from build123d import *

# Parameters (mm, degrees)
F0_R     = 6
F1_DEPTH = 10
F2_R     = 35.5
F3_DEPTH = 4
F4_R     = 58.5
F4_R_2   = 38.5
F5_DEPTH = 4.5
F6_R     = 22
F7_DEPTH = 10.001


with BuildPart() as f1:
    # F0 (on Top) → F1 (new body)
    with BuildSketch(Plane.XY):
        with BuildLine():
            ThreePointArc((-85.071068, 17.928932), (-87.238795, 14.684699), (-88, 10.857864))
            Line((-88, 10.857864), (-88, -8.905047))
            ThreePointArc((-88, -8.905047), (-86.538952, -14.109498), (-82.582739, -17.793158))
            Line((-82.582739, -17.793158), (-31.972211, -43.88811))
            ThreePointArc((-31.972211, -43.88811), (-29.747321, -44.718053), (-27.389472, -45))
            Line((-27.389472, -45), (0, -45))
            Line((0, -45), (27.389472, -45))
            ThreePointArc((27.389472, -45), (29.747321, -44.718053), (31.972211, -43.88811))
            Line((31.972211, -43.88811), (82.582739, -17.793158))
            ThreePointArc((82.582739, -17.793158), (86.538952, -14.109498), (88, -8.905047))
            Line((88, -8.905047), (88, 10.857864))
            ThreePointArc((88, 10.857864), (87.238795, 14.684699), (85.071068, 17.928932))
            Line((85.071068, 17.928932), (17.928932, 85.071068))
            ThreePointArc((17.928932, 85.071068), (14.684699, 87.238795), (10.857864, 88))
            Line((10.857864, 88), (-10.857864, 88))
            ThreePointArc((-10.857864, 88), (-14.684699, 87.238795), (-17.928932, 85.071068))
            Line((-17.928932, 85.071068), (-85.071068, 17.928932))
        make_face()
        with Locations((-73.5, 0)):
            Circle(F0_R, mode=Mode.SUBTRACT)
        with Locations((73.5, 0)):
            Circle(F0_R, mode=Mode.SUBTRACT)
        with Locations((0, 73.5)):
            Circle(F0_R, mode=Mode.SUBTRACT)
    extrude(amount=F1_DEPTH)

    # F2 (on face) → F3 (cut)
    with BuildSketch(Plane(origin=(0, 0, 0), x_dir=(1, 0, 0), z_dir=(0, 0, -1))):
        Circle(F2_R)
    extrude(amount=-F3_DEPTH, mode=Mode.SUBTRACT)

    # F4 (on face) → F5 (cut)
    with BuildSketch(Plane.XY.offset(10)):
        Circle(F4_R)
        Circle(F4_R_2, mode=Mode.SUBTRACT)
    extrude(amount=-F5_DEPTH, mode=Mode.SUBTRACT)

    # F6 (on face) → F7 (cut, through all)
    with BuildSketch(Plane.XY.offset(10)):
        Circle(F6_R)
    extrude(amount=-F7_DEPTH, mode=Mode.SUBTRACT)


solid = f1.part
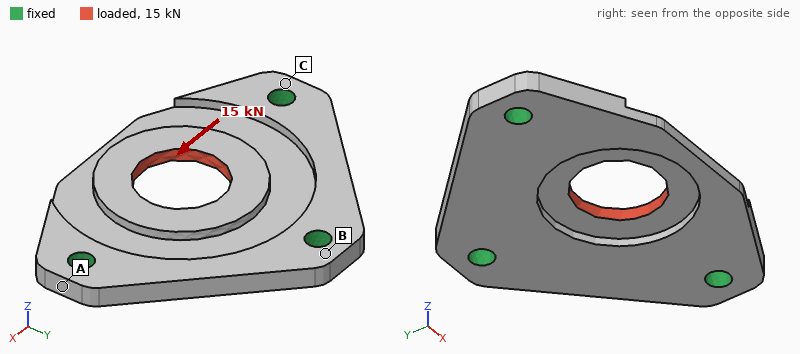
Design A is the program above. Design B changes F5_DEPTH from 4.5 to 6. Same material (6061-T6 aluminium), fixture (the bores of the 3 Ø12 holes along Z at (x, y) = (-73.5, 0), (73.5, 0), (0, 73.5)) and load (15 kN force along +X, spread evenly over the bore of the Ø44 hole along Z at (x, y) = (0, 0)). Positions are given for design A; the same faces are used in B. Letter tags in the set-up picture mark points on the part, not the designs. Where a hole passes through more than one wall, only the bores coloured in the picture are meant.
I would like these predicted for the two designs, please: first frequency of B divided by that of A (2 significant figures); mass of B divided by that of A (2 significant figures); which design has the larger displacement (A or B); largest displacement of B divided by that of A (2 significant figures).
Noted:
0.94
0.93
B
1.5
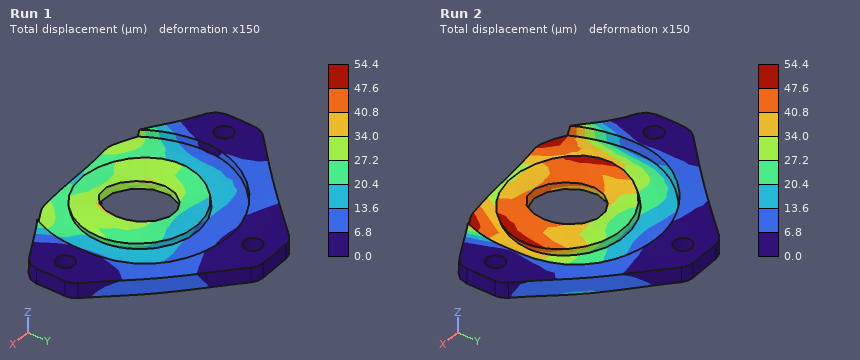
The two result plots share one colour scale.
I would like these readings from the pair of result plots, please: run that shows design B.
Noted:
Run 2
